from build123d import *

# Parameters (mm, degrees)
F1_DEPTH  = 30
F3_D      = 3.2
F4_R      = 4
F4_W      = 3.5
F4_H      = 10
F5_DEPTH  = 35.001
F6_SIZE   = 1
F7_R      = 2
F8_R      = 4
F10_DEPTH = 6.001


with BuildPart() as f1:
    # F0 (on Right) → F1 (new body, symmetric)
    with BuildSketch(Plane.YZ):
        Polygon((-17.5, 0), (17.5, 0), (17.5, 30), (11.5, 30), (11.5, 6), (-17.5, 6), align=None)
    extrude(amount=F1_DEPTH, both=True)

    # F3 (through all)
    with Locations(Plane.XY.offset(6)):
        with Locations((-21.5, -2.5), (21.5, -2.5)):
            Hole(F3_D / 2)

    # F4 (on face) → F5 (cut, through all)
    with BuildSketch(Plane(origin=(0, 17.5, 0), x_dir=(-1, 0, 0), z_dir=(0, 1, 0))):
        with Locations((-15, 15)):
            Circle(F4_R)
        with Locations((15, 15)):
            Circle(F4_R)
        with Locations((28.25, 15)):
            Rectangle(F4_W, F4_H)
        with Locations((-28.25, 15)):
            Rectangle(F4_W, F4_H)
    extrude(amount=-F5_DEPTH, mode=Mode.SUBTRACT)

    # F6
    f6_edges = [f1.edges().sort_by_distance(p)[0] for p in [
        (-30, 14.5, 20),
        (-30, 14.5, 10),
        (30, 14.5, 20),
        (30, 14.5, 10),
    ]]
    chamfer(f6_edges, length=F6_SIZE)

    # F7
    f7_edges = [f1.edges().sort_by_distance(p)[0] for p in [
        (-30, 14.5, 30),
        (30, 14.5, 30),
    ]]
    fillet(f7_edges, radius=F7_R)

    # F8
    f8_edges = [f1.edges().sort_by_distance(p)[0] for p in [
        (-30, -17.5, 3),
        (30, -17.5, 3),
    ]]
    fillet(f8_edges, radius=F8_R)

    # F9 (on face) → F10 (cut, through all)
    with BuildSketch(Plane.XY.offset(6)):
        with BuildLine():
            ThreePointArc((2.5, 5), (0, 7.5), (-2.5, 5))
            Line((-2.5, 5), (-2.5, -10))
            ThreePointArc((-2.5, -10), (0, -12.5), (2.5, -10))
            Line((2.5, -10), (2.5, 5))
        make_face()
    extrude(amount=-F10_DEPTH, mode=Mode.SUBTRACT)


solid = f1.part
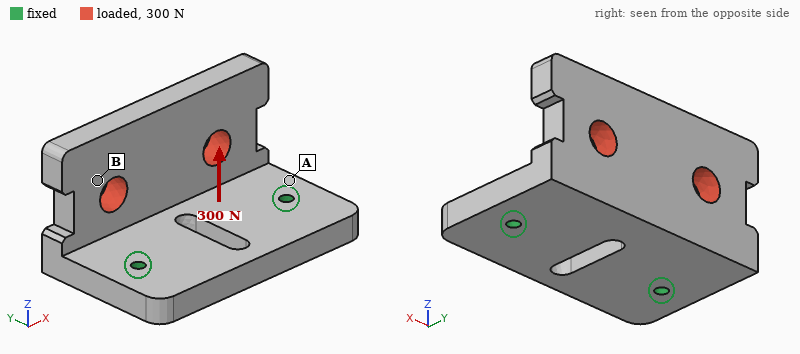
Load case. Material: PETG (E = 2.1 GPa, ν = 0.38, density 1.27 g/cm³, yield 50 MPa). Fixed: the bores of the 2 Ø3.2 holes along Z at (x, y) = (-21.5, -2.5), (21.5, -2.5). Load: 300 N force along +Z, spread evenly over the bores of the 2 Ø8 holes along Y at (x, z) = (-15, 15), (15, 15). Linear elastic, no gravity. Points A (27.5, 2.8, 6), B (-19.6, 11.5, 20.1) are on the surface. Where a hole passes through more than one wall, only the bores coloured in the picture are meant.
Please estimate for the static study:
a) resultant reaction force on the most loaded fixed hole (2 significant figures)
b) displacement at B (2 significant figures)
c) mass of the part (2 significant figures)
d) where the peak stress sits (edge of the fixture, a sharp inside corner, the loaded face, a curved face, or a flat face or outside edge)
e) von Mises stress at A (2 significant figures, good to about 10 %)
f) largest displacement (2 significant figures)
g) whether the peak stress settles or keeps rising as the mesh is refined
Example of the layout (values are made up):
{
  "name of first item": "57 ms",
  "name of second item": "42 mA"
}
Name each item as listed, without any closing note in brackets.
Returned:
{
  "resultant reaction force on the most loaded fixed hole": "150 N",
  "displacement at B": "0.58 mm",
  "mass of the part": "25 g",
  "where the peak stress sits": "edge of the fixture",
  "von Mises stress at A": "11 MPa",
  "largest displacement": "0.90 mm",
  "whether the peak stress settles or keeps rising as the mesh is refined": "keeps rising"
}
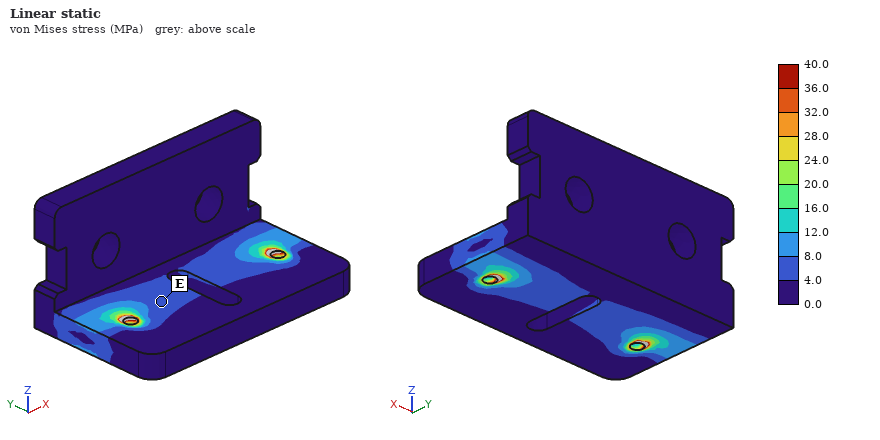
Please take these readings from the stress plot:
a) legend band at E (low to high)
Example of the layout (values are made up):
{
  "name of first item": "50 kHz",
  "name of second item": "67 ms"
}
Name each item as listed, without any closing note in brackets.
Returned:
{
  "legend band at E": "4.0 to 8.0 MPa"
}
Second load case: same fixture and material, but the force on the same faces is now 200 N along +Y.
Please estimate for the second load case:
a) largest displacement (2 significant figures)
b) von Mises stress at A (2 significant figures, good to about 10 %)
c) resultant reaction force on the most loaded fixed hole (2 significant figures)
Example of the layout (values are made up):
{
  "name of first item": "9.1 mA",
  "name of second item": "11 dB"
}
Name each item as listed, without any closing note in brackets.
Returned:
{
  "largest displacement": "0.78 mm",
  "von Mises stress at A": "7.2 MPa",
  "resultant reaction force on the most loaded fixed hole": "100 N"
}
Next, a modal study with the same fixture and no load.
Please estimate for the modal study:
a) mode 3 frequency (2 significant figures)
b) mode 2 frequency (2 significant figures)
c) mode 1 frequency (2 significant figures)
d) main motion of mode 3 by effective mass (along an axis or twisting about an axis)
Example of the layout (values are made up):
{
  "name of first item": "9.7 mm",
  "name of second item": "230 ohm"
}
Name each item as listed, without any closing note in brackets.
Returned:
{
  "mode 3 frequency": "2000 Hz",
  "mode 2 frequency": "1400 Hz",
  "mode 1 frequency": "740 Hz",
  "main motion of mode 3 by effective mass": "along Z"
}
